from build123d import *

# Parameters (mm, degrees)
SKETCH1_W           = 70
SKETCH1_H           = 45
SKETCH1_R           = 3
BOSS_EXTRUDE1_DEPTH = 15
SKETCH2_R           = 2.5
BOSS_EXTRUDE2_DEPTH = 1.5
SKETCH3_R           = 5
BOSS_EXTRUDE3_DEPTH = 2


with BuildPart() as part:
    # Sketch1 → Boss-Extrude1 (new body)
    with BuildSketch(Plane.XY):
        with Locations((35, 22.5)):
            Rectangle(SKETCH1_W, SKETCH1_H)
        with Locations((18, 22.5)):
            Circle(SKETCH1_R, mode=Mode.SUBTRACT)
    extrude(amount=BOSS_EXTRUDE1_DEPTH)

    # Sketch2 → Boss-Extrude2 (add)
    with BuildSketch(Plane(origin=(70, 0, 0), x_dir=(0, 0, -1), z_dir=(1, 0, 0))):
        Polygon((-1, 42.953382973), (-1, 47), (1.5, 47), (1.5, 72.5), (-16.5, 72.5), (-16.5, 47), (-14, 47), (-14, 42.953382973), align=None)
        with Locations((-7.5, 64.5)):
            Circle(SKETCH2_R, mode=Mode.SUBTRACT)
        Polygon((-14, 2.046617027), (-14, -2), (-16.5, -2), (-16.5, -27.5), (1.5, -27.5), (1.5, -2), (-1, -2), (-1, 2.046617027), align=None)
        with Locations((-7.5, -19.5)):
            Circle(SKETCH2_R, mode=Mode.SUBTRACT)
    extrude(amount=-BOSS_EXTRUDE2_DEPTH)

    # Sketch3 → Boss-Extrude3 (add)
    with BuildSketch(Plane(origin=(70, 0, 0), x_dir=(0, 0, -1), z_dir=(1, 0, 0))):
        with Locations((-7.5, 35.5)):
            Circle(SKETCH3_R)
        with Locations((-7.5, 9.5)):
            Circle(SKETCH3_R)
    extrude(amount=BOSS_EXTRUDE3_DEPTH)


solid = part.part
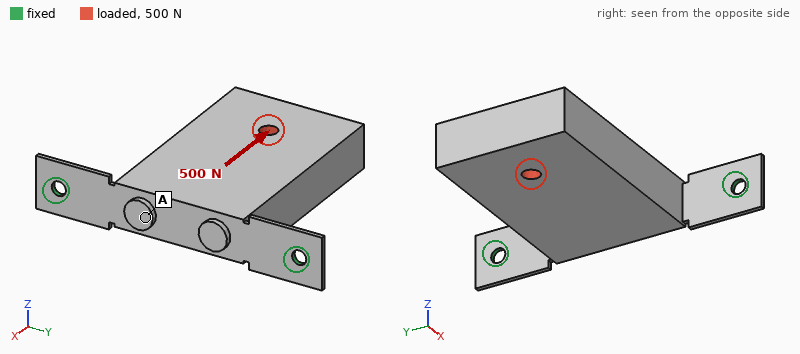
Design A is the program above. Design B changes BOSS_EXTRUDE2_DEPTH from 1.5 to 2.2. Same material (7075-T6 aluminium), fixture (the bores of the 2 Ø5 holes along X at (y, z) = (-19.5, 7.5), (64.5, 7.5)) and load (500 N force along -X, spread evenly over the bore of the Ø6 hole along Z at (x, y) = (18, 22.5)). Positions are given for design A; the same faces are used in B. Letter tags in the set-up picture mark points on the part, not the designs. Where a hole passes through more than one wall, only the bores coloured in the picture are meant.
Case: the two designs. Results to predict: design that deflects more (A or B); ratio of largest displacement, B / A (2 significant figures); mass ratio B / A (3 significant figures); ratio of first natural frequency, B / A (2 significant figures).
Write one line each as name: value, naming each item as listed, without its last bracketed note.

design that deflects more: A
ratio of largest displacement, B / A: 0.36
mass ratio B / A: 1.01
ratio of first natural frequency, B / A: 1.7
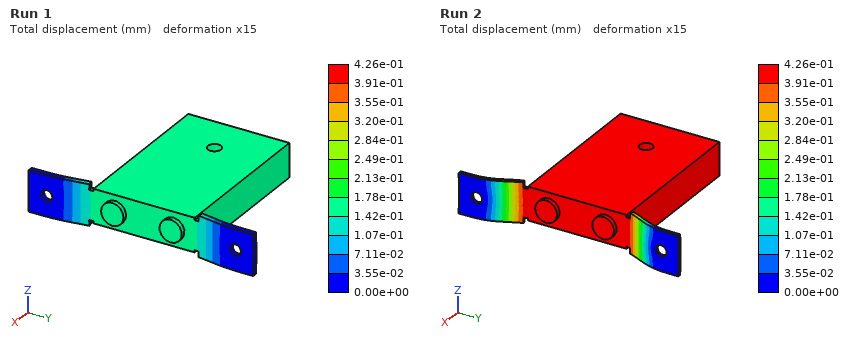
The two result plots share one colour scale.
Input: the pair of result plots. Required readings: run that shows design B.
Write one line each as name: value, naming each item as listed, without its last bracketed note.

run that shows design B: Run 1
